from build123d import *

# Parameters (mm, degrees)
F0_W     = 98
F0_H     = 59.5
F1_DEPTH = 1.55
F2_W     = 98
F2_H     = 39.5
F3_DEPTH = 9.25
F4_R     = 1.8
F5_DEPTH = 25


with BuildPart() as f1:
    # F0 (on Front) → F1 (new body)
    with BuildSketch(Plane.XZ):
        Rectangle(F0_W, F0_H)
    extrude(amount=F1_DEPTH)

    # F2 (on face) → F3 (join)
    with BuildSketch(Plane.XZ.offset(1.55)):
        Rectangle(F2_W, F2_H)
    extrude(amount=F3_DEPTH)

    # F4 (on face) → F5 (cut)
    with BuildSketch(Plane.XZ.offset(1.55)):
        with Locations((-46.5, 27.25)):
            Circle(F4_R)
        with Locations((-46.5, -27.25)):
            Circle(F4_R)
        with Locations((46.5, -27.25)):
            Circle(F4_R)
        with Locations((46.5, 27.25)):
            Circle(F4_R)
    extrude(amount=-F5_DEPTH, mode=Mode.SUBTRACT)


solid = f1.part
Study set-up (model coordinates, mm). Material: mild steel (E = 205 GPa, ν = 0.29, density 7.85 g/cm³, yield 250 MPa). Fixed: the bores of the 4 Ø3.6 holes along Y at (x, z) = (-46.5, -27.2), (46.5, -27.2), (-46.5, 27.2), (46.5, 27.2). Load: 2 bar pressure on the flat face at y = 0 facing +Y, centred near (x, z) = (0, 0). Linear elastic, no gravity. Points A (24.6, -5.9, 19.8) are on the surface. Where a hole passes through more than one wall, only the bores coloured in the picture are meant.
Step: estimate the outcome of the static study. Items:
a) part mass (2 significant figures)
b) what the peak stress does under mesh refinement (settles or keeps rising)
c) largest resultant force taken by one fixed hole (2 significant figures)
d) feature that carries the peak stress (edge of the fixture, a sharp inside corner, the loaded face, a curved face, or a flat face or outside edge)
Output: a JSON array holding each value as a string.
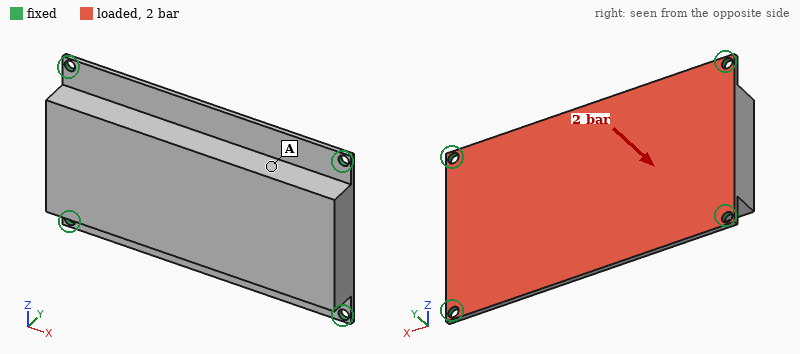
["350 g", "keeps rising", "430 N", "edge of the fixture"]
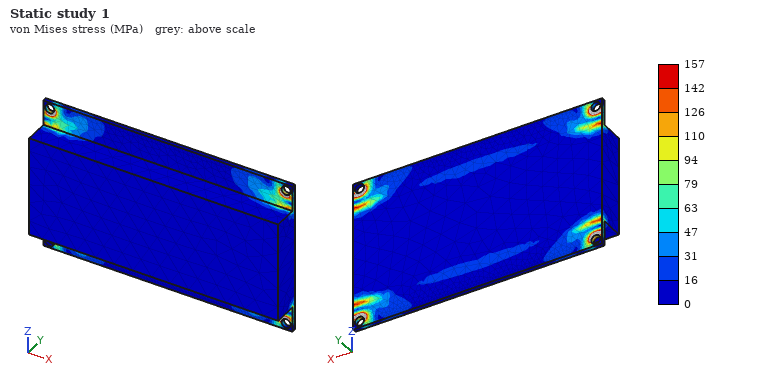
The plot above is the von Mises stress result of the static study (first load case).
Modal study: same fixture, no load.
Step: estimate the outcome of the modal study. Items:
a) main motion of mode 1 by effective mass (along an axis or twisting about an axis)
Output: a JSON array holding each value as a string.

["along Y"]
